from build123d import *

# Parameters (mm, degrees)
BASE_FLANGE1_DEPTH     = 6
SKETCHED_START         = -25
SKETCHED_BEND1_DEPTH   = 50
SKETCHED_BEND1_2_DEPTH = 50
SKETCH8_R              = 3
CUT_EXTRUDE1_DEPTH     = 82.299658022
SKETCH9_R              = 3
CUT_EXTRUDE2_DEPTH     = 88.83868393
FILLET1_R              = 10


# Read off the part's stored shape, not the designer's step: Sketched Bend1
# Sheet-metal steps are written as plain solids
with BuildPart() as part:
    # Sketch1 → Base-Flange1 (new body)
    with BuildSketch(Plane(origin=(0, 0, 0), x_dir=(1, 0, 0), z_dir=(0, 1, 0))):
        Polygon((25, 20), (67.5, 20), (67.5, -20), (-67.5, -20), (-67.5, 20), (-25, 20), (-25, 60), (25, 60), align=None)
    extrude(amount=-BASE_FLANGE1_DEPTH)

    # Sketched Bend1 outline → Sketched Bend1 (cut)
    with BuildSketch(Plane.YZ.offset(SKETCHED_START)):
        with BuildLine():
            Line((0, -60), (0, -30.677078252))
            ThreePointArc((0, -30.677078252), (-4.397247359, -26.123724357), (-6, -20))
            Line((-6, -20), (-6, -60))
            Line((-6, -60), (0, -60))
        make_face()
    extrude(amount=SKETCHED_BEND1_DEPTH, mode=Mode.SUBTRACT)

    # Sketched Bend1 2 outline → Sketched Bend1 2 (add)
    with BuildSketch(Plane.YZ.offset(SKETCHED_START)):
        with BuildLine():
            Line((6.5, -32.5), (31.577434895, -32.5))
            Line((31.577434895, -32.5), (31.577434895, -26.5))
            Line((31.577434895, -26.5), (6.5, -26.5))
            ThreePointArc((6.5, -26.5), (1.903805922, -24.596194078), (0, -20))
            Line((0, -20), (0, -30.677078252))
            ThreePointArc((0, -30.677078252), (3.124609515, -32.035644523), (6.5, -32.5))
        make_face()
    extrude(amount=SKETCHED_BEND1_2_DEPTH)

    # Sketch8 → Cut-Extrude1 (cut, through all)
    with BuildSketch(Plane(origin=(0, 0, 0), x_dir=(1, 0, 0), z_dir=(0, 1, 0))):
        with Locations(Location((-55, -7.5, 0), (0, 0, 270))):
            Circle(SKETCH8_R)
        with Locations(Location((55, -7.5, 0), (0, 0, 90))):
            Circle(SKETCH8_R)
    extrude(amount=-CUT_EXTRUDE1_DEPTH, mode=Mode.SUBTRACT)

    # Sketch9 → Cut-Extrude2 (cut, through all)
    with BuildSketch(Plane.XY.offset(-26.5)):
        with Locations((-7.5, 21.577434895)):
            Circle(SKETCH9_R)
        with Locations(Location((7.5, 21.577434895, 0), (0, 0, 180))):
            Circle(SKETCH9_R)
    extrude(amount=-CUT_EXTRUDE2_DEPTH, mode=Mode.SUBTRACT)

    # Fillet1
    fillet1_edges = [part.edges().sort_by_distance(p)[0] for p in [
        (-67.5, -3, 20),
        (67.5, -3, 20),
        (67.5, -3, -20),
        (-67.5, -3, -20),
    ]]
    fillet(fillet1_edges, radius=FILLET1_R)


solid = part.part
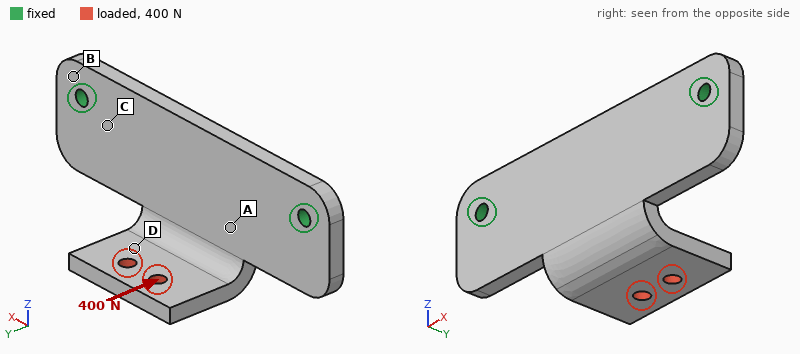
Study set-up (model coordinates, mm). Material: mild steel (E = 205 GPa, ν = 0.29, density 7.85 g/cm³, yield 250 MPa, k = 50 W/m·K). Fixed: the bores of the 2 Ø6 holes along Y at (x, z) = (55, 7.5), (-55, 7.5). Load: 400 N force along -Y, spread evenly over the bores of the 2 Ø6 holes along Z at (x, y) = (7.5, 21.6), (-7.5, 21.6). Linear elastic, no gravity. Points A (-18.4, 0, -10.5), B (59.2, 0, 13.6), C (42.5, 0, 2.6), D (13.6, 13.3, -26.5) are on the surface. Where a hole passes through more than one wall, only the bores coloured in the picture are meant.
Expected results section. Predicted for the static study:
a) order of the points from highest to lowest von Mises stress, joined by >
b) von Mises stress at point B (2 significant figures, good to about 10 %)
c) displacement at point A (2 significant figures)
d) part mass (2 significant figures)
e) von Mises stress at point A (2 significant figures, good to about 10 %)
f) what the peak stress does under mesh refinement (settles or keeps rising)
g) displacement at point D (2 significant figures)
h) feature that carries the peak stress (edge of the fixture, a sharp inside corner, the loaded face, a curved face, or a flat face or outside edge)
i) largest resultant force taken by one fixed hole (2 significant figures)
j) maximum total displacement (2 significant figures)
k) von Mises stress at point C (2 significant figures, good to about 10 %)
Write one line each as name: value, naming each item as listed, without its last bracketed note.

order of the points from highest to lowest von Mises stress, joined by >: C > A > B > D
von Mises stress at point B: 11 MPa
displacement at point A: 27 µm
part mass: 340 g
von Mises stress at point A: 20 MPa
what the peak stress does under mesh refinement: keeps rising
displacement at point D: 57 µm
feature that carries the peak stress: edge of the fixture
largest resultant force taken by one fixed hole: 200 N
maximum total displacement: 83 µm
von Mises stress at point C: 25 MPa
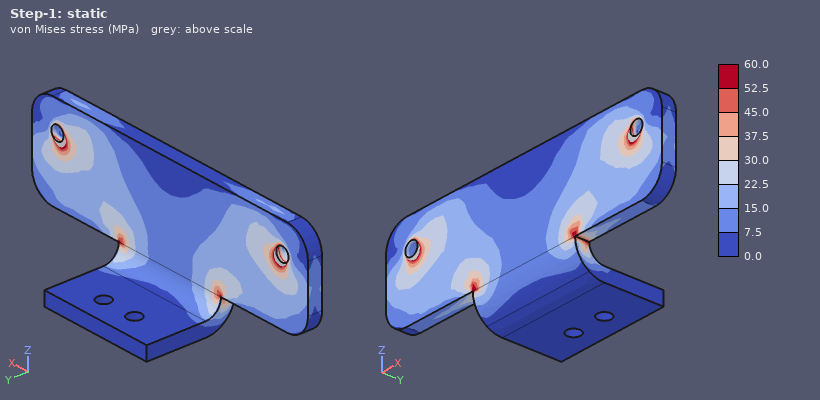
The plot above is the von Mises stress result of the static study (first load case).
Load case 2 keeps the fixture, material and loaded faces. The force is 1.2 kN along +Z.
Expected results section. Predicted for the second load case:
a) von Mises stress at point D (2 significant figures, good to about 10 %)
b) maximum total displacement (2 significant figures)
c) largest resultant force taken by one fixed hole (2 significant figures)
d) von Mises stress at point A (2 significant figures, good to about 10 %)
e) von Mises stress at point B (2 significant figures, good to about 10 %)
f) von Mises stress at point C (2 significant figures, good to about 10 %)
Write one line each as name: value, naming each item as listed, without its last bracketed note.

von Mises stress at point D: 36 MPa
maximum total displacement: 0.27 mm
largest resultant force taken by one fixed hole: 770 N
von Mises stress at point A: 66 MPa
von Mises stress at point B: 22 MPa
von Mises stress at point C: 62 MPa
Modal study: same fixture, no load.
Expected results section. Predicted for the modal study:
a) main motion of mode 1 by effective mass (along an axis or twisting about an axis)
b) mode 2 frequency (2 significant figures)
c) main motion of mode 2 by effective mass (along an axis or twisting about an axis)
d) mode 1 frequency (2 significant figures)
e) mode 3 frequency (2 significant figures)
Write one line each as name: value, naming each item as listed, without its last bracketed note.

main motion of mode 1 by effective mass: along Y
mode 2 frequency: 2400 Hz
main motion of mode 2 by effective mass: along Y
mode 1 frequency: 1200 Hz
mode 3 frequency: 2800 Hz
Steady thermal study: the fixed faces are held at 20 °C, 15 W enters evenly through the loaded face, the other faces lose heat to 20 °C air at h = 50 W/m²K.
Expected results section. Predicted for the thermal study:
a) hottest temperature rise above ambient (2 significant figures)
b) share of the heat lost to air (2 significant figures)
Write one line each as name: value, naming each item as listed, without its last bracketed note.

hottest temperature rise above ambient: 42 K
share of the heat lost to air: 68 %
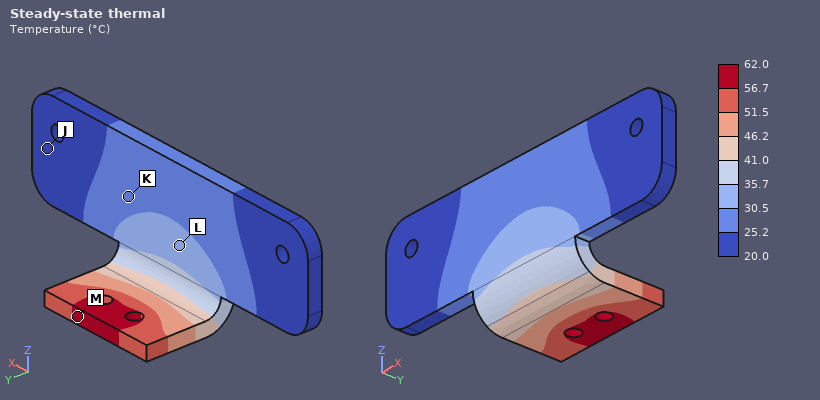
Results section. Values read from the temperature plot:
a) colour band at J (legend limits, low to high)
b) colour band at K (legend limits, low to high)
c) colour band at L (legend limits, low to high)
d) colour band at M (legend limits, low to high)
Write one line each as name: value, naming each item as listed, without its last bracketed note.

colour band at J: 20.0 to 25.2 °C
colour band at K: 25.2 to 30.5 °C
colour band at L: 30.5 to 35.7 °C
colour band at M: 56.7 to 62.0 °C
